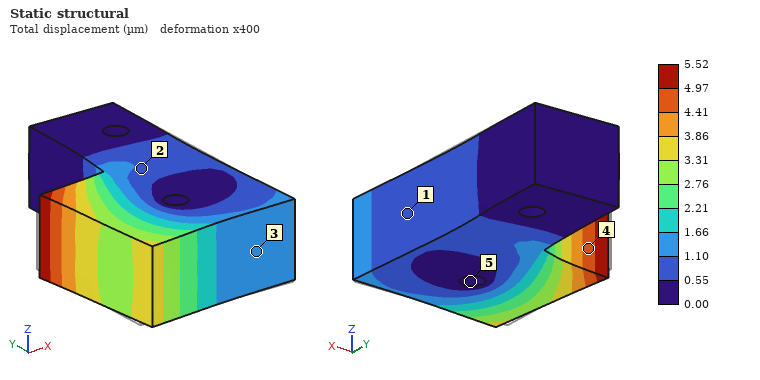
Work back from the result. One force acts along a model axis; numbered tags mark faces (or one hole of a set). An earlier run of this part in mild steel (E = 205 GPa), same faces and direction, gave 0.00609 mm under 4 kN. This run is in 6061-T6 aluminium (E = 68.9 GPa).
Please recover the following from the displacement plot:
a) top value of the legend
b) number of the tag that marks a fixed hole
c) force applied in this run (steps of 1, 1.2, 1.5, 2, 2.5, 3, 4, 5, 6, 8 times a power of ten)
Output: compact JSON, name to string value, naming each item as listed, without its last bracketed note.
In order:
{"top value of the legend": "5.52 µm", "number of the tag that marks a fixed hole": "5", "force applied in this run": "1.2 kN"}
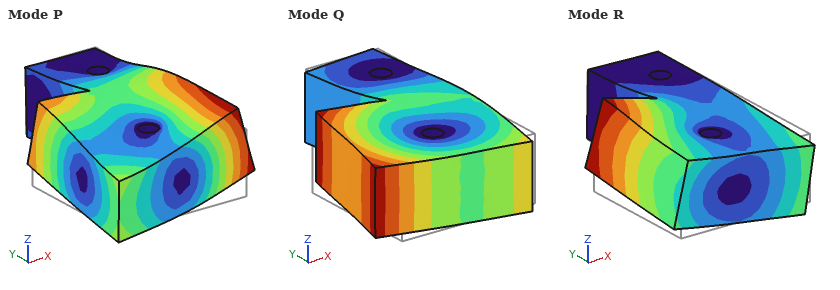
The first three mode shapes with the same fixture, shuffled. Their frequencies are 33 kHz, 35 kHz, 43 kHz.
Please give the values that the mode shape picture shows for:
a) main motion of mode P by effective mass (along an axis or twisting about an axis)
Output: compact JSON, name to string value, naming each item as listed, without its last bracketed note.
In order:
{"main motion of mode P by effective mass": "along Z"}
